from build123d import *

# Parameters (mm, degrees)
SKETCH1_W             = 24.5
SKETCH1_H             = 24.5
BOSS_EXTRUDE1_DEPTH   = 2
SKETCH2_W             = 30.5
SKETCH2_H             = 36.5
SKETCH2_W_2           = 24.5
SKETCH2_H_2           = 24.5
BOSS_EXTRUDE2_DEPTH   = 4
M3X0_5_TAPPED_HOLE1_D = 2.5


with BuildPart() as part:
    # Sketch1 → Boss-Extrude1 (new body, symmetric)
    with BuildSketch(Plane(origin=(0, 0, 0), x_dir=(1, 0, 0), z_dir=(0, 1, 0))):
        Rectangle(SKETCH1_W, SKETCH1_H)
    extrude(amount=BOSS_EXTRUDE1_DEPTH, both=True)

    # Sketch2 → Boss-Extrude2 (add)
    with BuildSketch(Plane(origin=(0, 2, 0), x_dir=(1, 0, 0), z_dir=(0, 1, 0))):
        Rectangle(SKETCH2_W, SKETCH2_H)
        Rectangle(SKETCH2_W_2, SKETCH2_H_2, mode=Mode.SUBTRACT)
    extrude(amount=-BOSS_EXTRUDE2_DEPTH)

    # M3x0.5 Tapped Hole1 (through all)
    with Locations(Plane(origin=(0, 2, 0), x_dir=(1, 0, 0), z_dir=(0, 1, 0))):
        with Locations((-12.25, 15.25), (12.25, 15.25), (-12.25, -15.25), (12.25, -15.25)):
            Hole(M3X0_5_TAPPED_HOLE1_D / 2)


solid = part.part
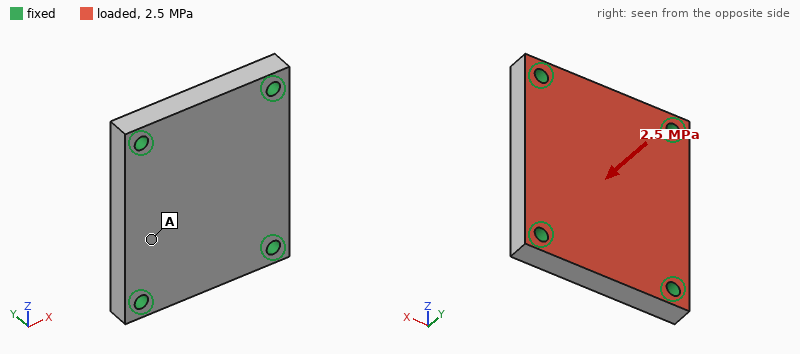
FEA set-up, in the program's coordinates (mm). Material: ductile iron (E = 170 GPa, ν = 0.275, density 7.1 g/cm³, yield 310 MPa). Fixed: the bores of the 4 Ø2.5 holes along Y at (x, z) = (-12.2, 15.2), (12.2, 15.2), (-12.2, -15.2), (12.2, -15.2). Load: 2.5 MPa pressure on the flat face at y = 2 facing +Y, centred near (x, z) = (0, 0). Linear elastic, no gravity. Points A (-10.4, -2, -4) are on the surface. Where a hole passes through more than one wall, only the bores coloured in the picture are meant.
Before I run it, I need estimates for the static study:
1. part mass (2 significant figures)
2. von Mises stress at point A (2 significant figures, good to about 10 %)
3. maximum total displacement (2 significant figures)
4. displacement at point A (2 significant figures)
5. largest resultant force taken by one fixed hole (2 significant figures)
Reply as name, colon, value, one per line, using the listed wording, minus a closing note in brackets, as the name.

part mass: 31 g
von Mises stress at point A: 36 MPa
maximum total displacement: 13 µm
displacement at point A: 9.5 µm
largest resultant force taken by one fixed hole: 680 N
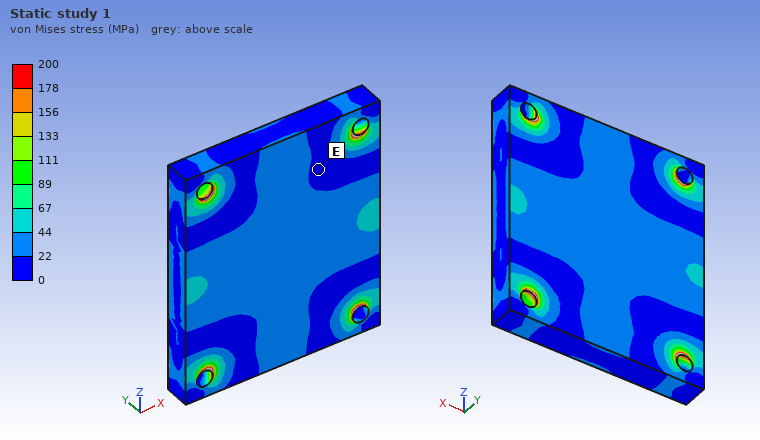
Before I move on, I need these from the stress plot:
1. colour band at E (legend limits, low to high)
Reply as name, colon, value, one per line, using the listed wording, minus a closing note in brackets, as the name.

colour band at E: 0 to 22 MPa
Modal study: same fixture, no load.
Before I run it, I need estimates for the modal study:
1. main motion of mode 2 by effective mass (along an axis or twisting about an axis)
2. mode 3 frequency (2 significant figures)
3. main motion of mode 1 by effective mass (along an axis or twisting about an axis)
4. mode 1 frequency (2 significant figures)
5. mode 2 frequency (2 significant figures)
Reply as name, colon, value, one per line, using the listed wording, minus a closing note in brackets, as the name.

main motion of mode 2 by effective mass: twisting about Z
mode 3 frequency: 30 kHz
main motion of mode 1 by effective mass: along Y
mode 1 frequency: 15 kHz
mode 2 frequency: 23 kHz
